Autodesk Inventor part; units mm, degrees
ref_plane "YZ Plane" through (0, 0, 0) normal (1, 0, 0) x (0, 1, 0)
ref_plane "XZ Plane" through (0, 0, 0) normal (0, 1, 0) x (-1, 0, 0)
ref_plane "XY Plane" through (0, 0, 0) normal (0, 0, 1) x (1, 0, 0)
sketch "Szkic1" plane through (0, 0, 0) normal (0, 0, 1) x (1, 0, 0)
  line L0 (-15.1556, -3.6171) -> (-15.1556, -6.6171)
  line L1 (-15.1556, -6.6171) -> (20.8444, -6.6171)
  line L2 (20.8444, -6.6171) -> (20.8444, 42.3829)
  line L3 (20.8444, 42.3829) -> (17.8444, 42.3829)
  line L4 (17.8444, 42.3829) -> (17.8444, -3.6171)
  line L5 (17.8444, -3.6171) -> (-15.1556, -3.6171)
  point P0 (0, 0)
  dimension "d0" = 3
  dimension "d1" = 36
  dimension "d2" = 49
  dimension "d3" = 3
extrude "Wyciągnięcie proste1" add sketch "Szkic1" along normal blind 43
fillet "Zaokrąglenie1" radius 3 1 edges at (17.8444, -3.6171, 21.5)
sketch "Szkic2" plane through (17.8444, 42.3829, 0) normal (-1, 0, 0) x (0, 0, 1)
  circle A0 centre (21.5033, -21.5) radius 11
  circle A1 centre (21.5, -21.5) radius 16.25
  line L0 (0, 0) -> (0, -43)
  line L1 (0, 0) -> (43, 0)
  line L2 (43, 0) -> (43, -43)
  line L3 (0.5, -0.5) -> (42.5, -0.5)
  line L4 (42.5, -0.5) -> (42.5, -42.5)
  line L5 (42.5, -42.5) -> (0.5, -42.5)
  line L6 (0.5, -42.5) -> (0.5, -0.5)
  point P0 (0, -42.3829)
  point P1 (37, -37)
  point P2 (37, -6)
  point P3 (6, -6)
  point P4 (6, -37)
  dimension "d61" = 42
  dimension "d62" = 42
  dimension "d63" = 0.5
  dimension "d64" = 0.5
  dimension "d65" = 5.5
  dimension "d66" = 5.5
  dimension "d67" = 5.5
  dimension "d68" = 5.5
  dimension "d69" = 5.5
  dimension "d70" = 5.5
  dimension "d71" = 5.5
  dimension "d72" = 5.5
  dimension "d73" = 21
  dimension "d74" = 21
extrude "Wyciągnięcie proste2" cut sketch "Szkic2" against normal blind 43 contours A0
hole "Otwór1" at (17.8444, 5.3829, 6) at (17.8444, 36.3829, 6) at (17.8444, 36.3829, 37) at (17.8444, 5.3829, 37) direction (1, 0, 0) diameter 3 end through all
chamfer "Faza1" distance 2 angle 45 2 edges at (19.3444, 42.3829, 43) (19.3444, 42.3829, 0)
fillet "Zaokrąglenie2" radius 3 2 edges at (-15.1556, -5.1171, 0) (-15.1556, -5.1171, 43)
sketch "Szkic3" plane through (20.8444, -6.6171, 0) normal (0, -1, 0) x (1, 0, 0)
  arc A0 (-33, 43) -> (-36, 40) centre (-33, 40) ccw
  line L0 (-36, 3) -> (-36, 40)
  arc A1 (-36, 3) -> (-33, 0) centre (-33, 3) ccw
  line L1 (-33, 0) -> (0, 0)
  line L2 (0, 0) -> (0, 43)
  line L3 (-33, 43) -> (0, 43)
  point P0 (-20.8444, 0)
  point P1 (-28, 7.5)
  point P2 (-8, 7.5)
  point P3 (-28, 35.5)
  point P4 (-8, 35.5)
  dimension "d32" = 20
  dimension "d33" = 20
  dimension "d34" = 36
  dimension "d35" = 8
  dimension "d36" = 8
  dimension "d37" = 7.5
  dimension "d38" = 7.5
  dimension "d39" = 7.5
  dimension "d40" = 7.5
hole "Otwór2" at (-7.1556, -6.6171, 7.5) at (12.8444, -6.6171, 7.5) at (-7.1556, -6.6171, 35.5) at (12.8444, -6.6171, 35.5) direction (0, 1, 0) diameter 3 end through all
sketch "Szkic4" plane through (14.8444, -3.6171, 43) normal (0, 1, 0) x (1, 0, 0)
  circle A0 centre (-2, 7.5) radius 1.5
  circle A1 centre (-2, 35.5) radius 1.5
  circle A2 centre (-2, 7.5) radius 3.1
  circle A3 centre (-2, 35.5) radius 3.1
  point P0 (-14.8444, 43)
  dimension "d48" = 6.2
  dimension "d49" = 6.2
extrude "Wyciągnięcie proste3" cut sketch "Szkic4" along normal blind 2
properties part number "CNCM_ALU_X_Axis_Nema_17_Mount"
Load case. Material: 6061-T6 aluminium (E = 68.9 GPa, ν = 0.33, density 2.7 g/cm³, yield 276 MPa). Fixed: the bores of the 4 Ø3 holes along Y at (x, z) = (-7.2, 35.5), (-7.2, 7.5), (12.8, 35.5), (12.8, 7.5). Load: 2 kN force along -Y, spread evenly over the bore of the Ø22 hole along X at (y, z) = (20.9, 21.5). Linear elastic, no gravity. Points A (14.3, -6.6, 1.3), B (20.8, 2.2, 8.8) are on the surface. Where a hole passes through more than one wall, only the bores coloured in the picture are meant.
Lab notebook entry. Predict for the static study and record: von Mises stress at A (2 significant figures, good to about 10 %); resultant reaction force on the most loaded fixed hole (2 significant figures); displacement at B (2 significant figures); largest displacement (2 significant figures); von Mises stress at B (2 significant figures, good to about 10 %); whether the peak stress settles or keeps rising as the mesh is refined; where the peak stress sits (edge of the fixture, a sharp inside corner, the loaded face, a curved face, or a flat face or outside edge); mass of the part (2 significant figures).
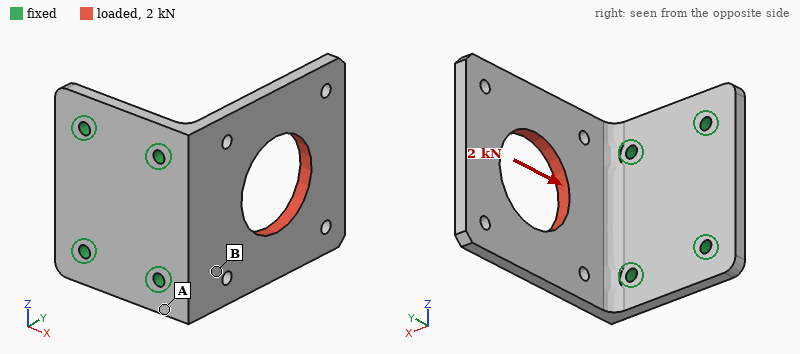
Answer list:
90 MPa
1.1 kN
0.071 mm
0.33 mm
29 MPa
keeps rising
edge of the fixture
25 g
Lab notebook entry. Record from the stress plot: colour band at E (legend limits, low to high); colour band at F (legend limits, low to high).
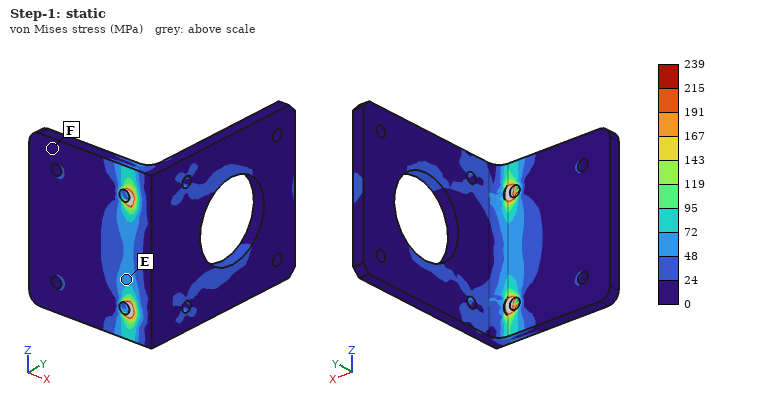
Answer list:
48 to 72 MPa
0 to 24 MPa
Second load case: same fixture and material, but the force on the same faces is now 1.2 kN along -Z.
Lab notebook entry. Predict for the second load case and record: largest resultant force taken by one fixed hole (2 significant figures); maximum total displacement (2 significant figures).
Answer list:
1.2 kN
0.18 mm
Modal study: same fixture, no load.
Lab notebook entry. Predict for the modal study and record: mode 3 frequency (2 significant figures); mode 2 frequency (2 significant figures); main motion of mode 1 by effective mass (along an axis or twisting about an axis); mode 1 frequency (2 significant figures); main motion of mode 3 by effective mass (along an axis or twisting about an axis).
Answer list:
4900 Hz
2400 Hz
along X
970 Hz
along Z
